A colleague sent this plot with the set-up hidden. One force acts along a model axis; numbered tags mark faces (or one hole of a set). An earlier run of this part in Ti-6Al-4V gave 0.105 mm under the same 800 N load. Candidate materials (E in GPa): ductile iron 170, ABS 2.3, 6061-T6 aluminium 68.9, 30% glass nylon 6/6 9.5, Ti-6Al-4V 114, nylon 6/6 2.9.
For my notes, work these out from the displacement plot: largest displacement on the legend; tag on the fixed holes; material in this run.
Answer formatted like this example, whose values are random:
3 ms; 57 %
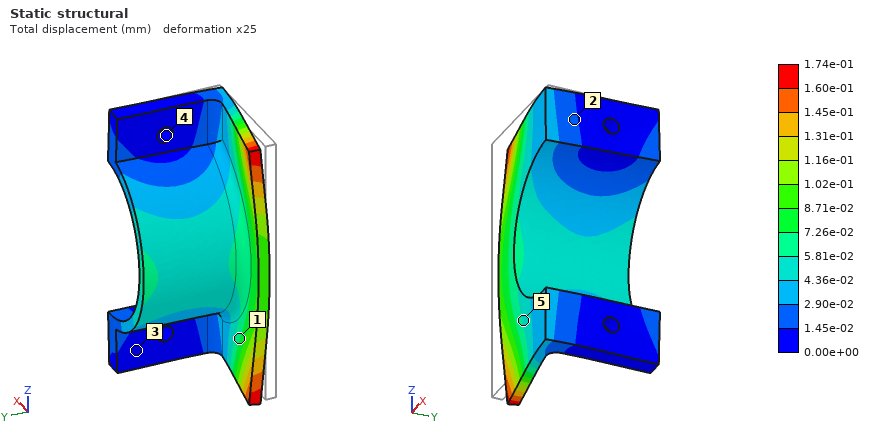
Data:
1.74e-01 mm; 4; 6061-T6 aluminium
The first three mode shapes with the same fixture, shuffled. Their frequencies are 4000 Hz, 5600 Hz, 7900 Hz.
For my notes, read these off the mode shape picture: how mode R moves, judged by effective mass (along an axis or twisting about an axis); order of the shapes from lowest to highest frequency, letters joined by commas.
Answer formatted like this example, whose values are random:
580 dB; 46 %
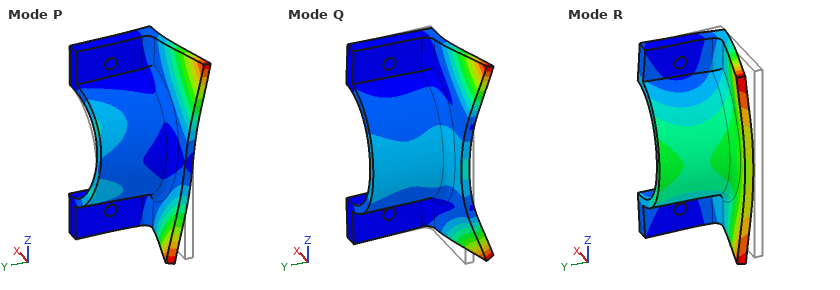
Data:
along Y; R, P, Q
